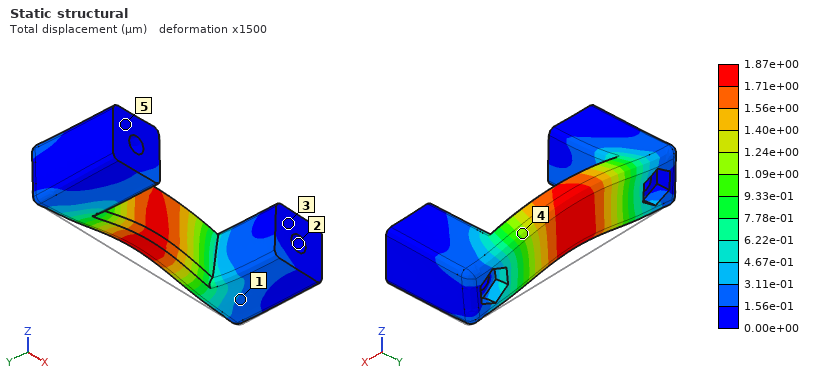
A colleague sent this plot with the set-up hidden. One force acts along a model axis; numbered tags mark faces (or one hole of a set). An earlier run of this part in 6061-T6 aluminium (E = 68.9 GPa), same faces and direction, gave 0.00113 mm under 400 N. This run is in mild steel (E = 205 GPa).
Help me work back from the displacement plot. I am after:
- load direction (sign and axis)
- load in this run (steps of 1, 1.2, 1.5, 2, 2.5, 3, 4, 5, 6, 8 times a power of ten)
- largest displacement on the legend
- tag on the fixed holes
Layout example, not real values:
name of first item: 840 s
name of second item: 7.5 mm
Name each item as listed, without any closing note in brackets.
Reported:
load direction: +Z
load in this run: 2 kN
largest displacement on the legend: 1.87e+00 µm
tag on the fixed holes: 2
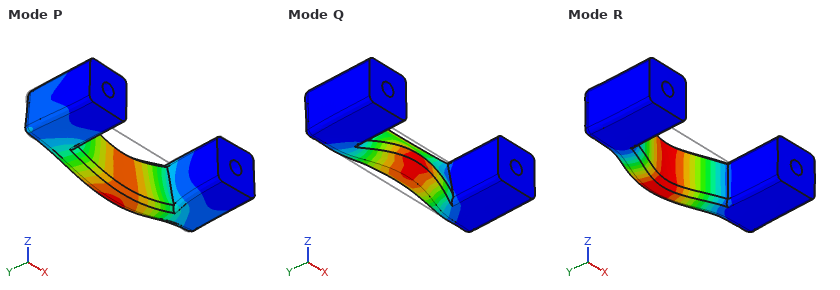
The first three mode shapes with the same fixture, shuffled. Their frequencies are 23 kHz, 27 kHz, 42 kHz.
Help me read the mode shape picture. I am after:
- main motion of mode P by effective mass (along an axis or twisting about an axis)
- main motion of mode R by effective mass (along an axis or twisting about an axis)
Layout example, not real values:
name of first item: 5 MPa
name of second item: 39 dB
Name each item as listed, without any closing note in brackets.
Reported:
main motion of mode P by effective mass: along Z
main motion of mode R by effective mass: along Y
